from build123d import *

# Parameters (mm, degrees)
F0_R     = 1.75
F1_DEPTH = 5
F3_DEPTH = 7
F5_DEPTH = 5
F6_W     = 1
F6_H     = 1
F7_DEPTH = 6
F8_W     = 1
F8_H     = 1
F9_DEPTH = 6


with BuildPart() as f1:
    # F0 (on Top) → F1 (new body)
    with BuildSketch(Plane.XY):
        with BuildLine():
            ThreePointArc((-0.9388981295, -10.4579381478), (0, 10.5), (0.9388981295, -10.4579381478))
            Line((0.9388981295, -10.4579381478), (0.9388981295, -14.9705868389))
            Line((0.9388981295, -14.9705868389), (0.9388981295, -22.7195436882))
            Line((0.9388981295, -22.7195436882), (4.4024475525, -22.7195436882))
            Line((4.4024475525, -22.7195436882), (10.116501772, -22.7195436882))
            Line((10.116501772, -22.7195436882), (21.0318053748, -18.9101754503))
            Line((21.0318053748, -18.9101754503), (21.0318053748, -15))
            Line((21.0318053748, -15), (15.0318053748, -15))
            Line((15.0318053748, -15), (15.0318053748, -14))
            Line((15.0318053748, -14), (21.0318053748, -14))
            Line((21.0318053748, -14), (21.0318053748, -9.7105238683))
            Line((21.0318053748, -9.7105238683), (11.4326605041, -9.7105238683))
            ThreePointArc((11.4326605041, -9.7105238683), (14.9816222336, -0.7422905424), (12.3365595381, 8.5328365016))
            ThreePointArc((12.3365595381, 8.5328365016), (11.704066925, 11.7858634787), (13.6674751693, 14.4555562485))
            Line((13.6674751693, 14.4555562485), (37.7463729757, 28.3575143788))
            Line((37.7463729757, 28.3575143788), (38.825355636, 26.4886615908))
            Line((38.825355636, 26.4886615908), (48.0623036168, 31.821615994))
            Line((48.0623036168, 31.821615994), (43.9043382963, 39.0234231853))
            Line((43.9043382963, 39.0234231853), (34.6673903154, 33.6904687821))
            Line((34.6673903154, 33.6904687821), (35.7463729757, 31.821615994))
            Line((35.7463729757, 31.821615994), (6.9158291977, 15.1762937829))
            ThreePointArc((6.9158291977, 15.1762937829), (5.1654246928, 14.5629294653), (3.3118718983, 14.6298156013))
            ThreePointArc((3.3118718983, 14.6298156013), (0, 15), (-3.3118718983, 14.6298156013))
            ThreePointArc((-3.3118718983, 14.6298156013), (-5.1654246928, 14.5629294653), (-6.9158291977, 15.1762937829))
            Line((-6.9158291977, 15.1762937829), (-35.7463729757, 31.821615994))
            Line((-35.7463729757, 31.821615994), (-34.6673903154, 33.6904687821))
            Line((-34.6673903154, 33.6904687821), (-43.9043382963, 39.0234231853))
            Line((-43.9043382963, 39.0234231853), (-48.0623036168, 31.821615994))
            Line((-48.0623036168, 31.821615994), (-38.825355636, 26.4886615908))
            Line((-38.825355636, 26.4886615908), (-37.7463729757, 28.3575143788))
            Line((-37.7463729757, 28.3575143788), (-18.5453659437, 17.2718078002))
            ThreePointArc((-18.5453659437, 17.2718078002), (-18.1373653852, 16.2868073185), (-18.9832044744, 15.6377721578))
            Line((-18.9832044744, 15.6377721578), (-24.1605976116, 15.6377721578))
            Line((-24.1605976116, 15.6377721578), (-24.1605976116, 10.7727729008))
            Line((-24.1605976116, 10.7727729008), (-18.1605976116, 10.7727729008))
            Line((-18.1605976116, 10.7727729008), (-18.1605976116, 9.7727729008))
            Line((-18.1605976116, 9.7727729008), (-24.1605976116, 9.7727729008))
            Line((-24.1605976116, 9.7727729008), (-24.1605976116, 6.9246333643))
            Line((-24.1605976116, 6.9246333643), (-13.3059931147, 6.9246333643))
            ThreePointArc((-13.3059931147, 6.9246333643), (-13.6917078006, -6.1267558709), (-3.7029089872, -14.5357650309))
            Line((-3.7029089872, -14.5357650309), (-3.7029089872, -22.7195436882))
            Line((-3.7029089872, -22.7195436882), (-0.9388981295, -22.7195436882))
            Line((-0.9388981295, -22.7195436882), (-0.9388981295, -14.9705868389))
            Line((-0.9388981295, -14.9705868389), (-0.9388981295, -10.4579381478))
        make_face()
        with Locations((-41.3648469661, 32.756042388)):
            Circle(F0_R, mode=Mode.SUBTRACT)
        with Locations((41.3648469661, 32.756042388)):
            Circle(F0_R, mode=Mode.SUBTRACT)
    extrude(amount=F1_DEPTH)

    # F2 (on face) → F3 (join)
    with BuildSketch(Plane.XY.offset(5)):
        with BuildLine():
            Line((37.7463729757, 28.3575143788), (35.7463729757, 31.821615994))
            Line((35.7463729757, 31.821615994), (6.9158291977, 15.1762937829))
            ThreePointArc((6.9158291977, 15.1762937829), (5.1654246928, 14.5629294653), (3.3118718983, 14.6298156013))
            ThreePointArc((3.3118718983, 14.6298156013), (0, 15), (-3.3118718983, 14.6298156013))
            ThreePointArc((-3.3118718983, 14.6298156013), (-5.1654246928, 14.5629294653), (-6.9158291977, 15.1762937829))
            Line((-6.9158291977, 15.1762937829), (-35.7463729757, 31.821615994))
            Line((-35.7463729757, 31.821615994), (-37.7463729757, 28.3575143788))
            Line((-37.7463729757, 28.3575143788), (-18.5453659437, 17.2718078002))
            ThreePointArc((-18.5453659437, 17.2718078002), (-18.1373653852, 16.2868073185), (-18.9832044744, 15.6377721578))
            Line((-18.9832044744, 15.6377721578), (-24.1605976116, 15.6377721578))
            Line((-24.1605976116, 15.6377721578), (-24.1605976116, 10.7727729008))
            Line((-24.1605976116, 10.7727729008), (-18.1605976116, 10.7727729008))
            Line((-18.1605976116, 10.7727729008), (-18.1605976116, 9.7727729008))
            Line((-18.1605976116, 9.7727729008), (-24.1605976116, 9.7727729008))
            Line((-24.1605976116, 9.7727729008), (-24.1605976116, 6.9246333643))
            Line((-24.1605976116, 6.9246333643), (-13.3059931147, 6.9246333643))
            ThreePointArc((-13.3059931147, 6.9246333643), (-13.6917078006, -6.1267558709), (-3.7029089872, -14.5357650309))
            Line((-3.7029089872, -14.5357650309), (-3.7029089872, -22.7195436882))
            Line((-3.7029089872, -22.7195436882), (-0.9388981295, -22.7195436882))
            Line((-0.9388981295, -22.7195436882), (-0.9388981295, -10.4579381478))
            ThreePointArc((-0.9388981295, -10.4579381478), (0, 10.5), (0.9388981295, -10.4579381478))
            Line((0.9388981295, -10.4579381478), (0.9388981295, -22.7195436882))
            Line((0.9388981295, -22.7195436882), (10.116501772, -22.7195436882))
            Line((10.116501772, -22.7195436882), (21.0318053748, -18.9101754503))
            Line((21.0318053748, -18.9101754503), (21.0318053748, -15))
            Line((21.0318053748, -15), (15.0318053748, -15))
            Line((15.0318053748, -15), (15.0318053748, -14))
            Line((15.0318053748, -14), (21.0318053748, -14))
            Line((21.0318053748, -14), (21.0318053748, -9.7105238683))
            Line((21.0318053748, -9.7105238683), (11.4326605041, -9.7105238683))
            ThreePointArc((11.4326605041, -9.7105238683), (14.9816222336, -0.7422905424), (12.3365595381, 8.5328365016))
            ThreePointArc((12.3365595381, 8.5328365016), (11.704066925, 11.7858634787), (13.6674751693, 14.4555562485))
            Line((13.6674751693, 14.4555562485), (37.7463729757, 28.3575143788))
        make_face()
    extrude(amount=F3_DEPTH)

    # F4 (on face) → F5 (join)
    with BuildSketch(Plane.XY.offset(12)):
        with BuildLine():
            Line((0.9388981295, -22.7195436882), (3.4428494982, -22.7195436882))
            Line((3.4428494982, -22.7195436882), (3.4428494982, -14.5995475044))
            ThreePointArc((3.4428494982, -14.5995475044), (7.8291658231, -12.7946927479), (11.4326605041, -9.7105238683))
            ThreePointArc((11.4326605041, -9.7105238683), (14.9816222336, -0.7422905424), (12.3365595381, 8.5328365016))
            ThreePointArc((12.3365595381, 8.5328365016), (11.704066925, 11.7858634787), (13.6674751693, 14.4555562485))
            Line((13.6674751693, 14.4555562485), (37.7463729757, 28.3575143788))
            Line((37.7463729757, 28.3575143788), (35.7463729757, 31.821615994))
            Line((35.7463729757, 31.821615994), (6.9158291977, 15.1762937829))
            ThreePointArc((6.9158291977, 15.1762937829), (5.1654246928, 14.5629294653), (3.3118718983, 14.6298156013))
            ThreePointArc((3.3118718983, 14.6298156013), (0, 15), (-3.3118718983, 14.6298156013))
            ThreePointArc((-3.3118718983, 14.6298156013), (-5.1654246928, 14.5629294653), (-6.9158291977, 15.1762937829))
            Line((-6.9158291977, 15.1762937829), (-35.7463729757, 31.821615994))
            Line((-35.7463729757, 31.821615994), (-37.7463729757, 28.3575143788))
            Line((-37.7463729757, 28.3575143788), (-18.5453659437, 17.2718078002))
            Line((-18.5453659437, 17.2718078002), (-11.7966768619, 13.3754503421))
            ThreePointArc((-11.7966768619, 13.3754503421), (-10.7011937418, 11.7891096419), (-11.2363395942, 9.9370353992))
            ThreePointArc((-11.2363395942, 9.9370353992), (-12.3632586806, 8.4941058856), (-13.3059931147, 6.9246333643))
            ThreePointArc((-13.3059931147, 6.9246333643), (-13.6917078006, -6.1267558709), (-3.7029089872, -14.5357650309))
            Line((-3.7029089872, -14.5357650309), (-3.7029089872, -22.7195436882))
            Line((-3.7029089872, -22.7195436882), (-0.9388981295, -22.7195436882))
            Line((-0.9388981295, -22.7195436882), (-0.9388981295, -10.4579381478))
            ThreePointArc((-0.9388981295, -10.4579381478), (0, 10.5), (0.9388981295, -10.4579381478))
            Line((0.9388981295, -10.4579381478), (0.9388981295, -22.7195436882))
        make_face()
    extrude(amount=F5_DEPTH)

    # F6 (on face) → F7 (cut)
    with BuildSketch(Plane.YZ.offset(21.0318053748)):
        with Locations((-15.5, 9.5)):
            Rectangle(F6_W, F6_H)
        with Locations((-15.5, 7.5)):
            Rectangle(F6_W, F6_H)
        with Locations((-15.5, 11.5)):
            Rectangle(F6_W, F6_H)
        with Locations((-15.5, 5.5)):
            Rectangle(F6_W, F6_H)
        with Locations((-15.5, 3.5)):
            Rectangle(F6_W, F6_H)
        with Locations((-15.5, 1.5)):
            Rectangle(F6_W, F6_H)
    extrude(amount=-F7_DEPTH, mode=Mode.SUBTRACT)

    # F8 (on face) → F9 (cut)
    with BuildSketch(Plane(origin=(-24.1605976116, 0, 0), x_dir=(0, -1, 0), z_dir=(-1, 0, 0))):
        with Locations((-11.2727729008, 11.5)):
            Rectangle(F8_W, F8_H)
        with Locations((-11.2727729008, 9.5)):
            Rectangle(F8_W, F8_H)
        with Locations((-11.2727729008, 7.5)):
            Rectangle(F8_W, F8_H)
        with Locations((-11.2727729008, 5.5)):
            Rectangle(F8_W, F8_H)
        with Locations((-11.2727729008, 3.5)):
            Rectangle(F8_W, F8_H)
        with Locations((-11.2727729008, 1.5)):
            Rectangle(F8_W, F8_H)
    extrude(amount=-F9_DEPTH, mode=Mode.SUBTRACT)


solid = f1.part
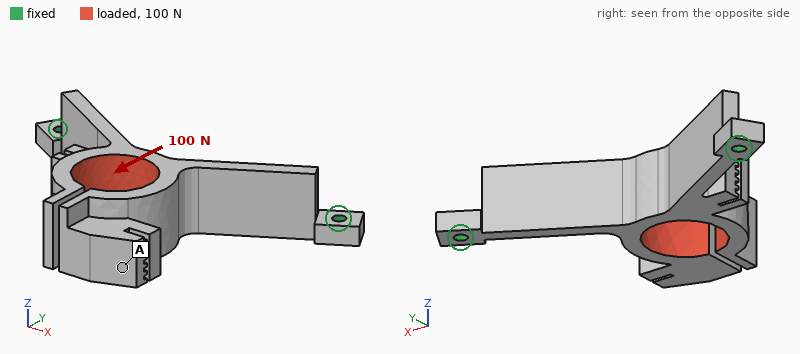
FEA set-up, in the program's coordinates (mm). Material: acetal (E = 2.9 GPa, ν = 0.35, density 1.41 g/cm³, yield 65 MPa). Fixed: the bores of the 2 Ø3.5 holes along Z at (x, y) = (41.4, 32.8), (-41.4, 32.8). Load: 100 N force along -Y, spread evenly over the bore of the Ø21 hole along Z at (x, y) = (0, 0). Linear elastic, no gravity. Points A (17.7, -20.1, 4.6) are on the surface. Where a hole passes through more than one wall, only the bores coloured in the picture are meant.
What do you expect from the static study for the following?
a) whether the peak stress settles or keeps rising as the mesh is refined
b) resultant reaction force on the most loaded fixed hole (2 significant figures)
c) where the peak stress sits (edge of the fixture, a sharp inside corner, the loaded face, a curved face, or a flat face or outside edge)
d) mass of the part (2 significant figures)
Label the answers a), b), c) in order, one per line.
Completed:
a) keeps rising
b) 91 N
c) a sharp inside corner
d) 22 g
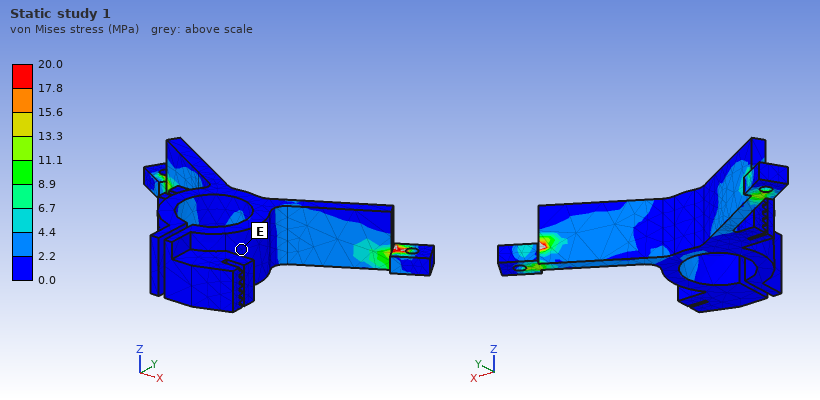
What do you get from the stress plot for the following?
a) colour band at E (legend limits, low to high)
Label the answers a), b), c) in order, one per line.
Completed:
a) 0.0 to 2.2 MPa
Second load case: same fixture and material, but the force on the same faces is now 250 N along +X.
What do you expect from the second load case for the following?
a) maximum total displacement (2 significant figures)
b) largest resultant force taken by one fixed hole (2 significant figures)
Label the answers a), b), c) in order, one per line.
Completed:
a) 1.4 mm
b) 170 N
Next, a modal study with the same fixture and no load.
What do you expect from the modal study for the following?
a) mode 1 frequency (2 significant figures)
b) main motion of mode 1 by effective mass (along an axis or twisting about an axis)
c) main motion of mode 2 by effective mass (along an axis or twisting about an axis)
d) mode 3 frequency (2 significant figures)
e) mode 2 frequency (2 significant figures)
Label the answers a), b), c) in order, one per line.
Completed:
a) 170 Hz
b) along Z
c) along X
d) 800 Hz
e) 440 Hz
